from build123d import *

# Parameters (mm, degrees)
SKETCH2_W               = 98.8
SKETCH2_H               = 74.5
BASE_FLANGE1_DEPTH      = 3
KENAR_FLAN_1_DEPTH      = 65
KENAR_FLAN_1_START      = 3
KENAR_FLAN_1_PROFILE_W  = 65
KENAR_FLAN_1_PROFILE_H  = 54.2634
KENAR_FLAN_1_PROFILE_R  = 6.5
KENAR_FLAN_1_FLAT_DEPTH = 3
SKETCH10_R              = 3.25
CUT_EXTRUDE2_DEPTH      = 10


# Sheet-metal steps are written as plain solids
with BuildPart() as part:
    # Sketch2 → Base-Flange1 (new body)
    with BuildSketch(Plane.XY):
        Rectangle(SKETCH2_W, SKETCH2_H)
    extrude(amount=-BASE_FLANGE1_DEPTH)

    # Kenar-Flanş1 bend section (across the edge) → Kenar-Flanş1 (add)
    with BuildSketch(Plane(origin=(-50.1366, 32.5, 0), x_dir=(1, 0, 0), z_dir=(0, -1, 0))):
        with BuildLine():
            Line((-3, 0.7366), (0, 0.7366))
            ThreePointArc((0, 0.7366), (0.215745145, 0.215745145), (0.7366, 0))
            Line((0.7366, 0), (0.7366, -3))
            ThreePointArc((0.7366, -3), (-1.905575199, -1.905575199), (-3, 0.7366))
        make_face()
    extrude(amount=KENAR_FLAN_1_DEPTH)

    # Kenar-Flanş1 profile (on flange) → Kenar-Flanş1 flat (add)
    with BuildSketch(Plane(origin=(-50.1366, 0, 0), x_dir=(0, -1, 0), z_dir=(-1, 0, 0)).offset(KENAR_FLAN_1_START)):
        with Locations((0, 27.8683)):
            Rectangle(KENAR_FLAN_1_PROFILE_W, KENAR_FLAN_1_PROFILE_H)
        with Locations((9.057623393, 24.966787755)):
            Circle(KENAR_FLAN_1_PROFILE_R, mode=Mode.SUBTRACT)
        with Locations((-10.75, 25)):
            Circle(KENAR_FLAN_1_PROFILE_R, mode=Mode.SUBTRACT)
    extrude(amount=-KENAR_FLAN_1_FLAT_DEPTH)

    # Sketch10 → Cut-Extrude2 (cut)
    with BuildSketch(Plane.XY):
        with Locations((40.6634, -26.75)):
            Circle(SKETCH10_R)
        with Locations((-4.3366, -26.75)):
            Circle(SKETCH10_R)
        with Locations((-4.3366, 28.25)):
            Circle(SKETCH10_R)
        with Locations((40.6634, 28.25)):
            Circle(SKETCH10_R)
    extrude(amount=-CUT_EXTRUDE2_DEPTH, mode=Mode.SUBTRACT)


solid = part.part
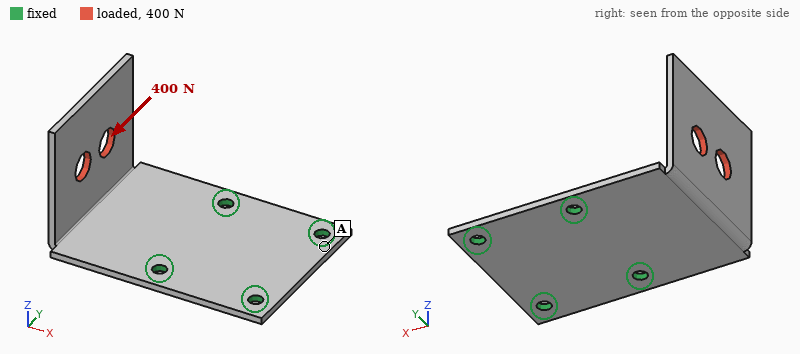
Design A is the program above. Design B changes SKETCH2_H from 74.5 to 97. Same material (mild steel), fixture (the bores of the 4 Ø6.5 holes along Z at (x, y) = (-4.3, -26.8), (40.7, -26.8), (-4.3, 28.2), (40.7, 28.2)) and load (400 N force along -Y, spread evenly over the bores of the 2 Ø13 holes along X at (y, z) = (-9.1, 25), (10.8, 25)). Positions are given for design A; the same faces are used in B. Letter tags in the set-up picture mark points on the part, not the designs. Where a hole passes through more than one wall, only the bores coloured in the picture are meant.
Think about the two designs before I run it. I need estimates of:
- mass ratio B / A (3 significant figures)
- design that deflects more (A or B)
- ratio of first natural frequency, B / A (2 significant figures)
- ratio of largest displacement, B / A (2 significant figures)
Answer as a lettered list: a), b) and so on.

a) 1.21
b) A
c) 1.1
d) 0.83
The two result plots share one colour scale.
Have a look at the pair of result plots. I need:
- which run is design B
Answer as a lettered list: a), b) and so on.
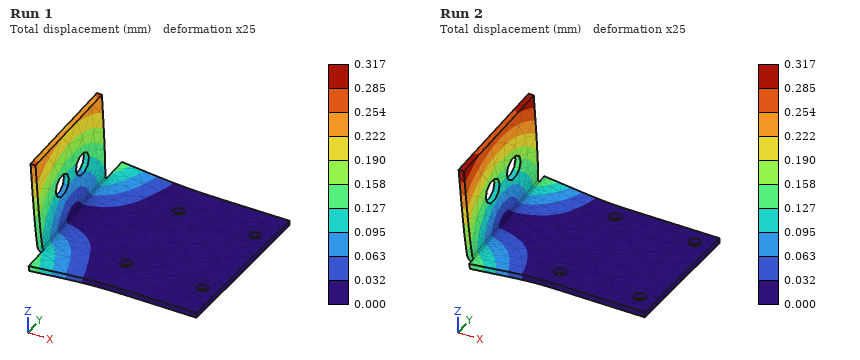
a) Run 1
